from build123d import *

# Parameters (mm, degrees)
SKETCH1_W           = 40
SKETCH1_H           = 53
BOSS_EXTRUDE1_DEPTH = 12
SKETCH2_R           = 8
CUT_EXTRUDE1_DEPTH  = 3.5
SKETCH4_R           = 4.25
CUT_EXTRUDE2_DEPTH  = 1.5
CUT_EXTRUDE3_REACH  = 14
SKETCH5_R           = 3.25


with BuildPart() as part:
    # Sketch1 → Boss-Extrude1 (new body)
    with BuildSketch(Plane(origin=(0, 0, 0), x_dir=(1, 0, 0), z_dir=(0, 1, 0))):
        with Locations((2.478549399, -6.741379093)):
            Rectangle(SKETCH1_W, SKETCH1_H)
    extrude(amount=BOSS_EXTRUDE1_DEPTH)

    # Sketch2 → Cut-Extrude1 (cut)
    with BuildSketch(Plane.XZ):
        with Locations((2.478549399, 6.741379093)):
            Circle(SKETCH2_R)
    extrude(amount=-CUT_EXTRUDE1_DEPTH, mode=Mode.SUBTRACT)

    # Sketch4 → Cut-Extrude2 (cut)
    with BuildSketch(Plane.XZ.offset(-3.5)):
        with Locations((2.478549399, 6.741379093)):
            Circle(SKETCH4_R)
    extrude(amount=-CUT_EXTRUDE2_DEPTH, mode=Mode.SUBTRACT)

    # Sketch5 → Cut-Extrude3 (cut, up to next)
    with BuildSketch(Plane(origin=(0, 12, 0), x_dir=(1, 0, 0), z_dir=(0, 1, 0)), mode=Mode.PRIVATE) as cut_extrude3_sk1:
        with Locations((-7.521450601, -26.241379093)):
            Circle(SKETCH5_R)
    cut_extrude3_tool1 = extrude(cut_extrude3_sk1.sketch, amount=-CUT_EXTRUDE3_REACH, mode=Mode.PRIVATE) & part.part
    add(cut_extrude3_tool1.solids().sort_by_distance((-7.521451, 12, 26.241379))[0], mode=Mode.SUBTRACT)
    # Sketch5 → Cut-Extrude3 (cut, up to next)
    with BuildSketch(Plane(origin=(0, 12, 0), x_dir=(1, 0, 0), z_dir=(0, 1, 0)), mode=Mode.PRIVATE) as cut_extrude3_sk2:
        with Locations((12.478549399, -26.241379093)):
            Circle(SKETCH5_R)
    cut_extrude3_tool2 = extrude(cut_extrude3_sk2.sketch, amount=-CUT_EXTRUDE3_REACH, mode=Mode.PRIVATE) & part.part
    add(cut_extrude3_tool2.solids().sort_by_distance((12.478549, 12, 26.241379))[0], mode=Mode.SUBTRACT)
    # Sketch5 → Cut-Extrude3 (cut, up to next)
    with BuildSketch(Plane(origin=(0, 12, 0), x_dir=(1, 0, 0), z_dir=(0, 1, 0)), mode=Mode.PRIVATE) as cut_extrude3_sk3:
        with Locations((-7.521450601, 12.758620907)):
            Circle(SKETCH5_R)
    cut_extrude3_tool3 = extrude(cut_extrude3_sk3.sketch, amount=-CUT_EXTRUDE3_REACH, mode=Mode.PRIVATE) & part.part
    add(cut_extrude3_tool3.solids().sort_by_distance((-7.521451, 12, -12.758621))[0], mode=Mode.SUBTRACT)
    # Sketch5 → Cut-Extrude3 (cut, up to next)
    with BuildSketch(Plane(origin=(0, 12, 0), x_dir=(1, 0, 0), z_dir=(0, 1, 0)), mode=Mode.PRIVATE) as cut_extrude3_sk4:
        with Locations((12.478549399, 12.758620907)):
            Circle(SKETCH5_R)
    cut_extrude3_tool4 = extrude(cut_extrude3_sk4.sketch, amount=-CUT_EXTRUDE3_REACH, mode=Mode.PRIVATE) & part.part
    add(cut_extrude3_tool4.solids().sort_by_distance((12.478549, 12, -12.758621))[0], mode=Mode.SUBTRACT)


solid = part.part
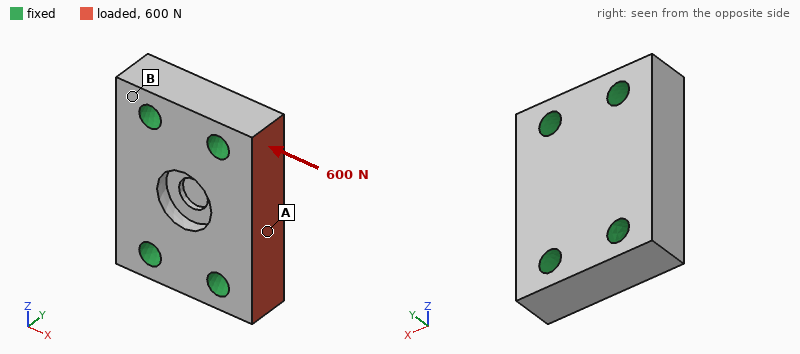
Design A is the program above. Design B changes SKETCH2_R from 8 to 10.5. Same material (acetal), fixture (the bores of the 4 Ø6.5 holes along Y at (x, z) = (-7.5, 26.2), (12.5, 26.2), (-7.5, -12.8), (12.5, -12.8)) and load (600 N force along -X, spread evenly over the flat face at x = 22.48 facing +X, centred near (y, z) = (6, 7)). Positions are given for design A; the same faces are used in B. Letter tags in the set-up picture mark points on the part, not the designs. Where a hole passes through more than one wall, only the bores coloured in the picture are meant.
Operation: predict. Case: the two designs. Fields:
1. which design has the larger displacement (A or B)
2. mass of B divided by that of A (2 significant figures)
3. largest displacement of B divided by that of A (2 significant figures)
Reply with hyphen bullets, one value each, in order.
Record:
- B
- 0.98
- 1.1
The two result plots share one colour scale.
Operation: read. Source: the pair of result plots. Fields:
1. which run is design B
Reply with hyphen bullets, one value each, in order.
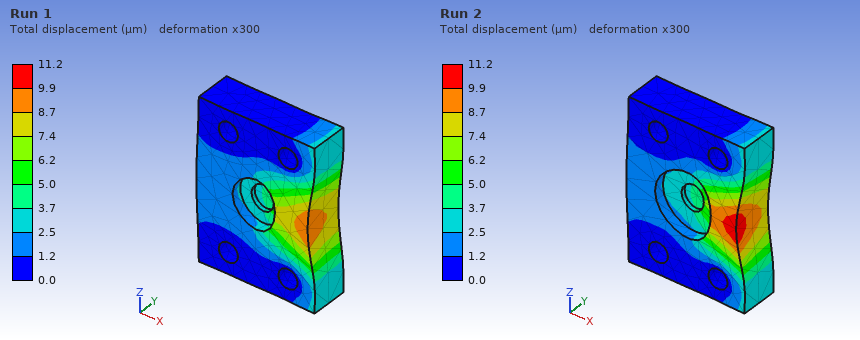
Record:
- Run 2
